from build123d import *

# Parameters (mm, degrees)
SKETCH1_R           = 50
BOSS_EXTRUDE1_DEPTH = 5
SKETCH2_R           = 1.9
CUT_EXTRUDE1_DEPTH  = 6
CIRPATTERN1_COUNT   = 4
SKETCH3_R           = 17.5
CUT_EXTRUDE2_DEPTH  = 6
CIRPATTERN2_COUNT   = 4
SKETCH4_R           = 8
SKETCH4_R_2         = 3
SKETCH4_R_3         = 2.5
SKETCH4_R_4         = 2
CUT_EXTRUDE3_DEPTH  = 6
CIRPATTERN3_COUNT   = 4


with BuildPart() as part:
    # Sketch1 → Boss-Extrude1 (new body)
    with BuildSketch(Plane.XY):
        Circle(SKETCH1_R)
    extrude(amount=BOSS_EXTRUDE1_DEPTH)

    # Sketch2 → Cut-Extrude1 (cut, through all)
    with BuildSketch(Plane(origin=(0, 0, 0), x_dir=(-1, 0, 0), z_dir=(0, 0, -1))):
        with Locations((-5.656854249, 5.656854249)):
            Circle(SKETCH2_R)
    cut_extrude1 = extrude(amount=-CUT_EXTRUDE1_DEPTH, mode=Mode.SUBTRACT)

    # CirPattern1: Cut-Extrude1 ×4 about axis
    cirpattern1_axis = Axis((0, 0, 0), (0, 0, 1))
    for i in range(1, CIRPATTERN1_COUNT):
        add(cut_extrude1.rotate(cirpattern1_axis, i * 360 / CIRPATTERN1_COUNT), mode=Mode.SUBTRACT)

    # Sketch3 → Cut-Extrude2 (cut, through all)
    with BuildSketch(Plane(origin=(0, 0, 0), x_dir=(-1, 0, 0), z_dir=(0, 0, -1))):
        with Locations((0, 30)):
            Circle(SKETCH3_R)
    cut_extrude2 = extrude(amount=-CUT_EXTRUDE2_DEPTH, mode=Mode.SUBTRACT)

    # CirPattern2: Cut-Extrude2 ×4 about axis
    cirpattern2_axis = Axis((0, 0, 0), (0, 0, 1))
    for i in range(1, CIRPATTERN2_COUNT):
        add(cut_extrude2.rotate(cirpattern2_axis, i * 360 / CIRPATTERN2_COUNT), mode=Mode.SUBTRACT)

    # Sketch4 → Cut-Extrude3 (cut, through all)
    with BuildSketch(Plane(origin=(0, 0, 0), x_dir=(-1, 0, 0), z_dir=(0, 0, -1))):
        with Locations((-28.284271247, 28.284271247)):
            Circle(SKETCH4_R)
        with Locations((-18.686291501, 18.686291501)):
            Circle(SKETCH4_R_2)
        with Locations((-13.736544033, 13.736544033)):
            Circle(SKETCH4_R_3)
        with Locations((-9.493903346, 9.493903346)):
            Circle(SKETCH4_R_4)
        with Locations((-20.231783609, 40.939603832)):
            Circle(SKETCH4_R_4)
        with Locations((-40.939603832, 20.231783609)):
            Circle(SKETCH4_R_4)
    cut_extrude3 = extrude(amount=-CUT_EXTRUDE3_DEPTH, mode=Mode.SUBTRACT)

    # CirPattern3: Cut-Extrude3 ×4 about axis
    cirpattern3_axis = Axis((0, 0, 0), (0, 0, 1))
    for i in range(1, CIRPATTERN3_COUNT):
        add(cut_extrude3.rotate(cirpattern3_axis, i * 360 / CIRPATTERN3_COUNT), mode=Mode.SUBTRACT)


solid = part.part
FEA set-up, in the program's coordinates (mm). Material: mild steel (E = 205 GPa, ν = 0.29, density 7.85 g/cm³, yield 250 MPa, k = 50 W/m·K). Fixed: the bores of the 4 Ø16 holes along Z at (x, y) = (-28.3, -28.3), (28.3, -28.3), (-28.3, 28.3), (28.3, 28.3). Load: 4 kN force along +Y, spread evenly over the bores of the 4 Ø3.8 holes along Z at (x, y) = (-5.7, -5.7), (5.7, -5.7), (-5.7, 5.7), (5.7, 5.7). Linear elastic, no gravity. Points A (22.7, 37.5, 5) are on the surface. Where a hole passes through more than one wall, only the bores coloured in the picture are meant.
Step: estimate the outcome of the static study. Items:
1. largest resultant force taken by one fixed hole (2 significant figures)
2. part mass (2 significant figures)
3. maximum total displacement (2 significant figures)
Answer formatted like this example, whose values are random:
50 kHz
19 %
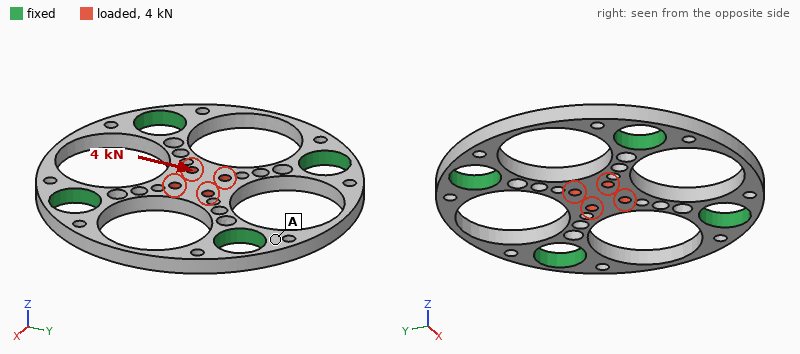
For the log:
1.3 kN
110 g
10 µm
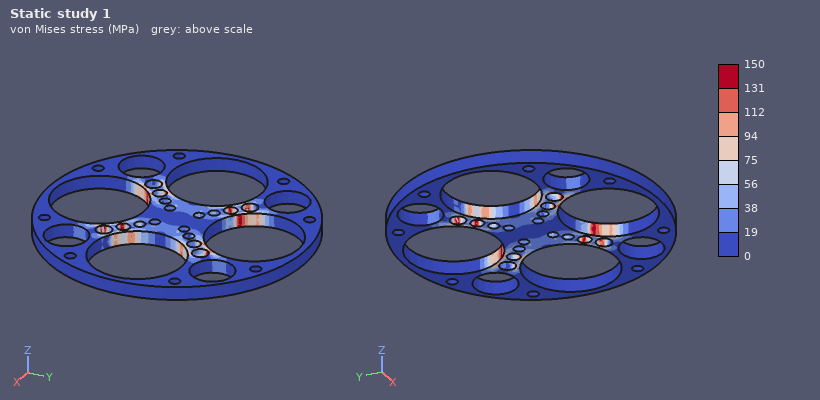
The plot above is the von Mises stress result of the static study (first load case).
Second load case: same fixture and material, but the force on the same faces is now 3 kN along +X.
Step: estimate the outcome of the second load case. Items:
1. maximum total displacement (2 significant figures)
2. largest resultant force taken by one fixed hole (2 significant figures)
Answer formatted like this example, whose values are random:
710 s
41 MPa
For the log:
7.7 µm
960 N
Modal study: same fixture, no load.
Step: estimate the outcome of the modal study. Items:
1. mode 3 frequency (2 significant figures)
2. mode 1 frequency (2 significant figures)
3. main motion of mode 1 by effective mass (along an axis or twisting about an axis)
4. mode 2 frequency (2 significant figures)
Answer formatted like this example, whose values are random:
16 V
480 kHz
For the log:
9200 Hz
6200 Hz
along Z
9200 Hz
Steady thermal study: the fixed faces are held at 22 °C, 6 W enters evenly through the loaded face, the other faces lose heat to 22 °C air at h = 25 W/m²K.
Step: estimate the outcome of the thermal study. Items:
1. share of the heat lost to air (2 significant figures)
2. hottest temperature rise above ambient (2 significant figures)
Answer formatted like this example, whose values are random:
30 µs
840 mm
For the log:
23 %
25 K
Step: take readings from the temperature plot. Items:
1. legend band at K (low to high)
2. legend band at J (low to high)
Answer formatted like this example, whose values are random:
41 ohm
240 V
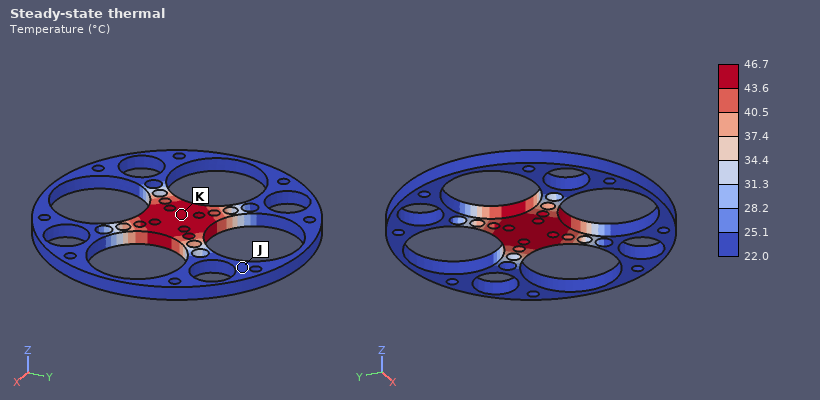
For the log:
43.6 to 46.7 °C
22.0 to 25.1 °C
